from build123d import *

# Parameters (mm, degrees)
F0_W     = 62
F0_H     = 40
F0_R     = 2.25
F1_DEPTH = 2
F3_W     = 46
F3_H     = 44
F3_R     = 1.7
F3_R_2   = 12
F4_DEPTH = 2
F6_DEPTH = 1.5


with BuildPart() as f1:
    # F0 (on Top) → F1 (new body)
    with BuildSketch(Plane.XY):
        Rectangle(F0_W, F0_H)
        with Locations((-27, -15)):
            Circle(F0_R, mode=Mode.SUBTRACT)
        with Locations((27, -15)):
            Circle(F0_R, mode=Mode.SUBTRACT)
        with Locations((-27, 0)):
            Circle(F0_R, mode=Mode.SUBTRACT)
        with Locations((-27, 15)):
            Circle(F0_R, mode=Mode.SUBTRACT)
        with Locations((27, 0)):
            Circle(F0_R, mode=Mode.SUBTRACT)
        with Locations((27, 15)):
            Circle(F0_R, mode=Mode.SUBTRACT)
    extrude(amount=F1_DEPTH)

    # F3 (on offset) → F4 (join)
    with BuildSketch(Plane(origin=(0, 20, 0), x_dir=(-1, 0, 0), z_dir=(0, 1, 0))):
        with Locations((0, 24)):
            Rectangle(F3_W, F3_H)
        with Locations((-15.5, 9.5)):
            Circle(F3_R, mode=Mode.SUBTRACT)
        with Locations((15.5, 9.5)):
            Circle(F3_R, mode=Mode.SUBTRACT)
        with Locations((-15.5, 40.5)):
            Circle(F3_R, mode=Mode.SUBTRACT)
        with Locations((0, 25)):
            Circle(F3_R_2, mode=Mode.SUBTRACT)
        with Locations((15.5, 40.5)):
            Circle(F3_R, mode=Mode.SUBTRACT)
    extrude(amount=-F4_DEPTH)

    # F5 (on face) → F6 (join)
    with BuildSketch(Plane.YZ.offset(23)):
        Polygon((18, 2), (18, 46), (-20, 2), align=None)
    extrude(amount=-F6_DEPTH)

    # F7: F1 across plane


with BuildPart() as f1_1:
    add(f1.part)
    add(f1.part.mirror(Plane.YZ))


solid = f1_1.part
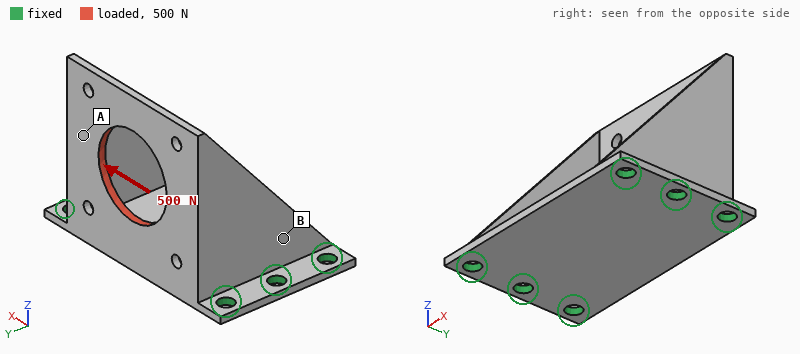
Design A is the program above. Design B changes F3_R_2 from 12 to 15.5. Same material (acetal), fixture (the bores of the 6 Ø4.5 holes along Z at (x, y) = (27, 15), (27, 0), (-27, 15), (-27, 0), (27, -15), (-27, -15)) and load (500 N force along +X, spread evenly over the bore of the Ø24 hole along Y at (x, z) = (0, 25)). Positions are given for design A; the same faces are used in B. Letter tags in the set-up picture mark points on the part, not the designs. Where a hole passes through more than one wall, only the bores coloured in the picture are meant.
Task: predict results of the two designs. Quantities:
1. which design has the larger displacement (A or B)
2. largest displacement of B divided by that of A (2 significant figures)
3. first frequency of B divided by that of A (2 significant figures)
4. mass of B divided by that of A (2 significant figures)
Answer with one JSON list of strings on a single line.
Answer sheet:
["B", "1.6", "1.0", "0.94"]
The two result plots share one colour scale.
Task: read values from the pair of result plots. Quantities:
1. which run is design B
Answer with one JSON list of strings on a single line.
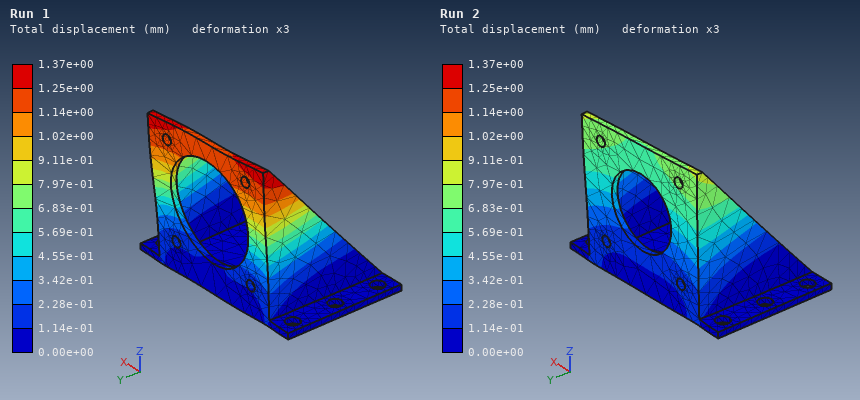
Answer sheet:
["Run 1"]
